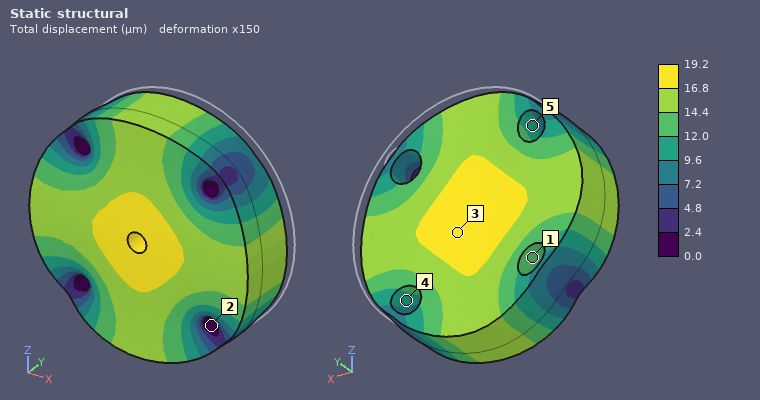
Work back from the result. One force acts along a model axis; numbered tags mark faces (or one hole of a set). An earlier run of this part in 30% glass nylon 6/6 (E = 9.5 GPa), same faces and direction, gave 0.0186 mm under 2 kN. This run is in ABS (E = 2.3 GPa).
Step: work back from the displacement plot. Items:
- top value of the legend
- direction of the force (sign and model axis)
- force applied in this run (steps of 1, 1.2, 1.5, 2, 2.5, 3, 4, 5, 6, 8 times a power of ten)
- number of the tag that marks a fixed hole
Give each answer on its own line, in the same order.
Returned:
19.2 µm
-Y
500 N
2
